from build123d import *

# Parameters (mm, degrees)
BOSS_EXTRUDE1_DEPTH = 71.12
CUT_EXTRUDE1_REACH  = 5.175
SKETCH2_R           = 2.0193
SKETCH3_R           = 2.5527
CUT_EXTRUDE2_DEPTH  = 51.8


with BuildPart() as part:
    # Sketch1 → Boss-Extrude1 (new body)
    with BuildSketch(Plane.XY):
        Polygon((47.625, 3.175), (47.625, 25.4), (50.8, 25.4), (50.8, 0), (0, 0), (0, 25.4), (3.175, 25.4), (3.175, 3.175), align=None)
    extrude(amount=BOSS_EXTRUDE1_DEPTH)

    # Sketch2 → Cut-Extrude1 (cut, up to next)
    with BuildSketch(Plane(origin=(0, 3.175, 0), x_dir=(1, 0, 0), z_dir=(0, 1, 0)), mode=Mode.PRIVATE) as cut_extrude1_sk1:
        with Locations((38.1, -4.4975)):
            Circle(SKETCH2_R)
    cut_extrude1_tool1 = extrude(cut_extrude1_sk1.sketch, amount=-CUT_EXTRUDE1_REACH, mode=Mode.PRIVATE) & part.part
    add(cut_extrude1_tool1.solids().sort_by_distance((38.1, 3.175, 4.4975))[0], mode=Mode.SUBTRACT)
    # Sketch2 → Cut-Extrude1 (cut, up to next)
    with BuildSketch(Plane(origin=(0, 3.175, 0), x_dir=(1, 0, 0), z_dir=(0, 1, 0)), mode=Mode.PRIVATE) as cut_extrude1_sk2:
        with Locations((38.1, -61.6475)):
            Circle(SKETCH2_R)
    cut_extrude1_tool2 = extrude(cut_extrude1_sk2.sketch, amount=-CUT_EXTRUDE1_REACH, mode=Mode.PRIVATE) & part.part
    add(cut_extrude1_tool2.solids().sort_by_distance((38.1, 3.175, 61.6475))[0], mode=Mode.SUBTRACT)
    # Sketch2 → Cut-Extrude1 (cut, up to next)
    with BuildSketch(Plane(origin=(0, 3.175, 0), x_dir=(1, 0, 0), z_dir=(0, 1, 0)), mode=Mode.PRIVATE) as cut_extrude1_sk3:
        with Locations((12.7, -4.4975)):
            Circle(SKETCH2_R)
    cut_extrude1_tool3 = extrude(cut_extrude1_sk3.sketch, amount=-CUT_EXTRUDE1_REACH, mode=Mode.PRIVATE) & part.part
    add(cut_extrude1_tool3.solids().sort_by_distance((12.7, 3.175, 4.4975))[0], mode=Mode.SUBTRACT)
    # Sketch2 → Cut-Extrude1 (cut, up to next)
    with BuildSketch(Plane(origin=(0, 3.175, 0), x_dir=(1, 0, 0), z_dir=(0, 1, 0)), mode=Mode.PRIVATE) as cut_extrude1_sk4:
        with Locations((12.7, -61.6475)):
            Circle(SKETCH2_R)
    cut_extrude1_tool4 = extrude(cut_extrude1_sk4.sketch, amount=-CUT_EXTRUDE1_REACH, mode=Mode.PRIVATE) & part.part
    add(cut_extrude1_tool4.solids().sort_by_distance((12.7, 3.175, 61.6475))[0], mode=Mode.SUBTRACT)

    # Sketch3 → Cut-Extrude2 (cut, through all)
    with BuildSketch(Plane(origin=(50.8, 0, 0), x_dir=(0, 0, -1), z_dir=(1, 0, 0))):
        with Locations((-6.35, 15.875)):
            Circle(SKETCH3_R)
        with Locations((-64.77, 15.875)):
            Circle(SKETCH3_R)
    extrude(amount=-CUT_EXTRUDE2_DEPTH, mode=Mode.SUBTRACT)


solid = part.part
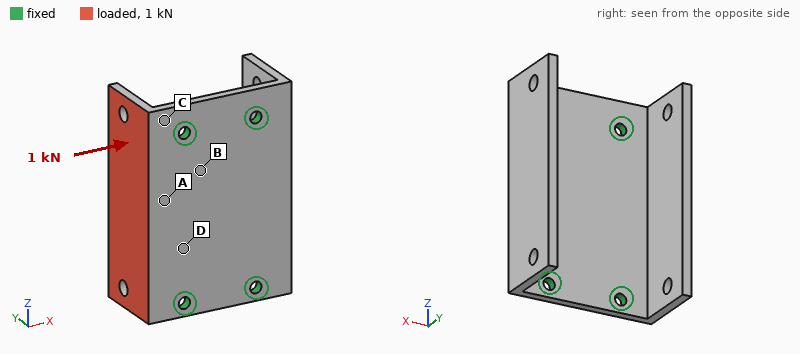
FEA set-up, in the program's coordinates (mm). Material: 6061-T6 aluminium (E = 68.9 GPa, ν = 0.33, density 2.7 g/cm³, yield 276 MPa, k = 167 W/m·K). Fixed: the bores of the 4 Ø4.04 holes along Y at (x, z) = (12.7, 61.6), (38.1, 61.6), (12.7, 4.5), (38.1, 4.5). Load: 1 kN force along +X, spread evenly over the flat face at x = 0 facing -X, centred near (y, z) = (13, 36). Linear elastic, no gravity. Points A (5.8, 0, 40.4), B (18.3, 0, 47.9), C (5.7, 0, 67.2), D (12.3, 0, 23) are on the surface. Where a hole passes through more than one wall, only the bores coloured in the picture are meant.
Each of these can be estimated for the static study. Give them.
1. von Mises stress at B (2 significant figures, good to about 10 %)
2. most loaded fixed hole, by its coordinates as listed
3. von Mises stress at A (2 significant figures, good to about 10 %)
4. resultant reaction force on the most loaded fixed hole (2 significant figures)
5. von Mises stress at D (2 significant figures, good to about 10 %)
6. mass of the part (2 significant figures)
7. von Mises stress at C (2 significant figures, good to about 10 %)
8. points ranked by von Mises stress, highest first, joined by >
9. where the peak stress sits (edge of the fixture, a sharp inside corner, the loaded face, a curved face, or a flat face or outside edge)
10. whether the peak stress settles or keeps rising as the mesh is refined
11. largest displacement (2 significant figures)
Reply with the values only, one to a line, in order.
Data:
25 MPa
(12.7, 61.6)
65 MPa
380 N
48 MPa
57 g
87 MPa
C > A > D > B
edge of the fixture
keeps rising
0.35 mm
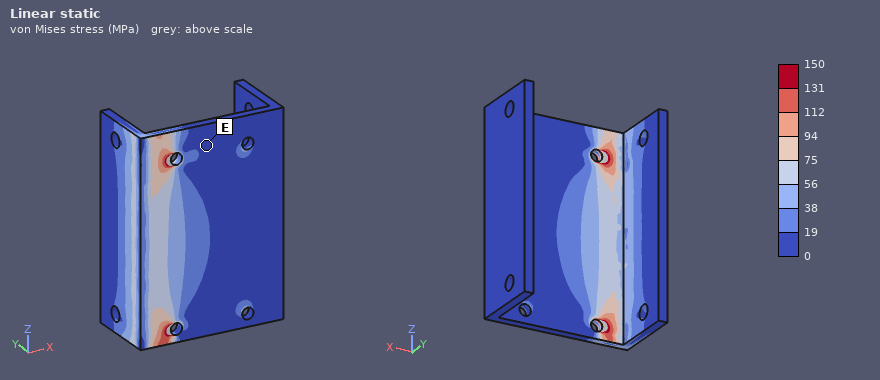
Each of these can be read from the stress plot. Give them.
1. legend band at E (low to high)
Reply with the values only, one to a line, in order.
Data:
0 to 19 MPa
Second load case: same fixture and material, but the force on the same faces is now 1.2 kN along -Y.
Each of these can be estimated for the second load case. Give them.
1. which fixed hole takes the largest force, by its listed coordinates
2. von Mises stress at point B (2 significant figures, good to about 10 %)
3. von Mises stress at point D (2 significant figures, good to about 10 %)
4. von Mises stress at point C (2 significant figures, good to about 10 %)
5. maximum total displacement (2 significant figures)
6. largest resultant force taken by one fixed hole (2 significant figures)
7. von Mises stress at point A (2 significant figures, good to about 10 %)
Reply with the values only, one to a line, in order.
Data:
(12.7, 61.6)
29 MPa
38 MPa
70 MPa
0.25 mm
760 N
36 MPa
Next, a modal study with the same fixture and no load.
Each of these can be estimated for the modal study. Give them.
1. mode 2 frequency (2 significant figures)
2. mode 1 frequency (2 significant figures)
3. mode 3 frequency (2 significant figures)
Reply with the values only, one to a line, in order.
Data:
2600 Hz
2500 Hz
4100 Hz
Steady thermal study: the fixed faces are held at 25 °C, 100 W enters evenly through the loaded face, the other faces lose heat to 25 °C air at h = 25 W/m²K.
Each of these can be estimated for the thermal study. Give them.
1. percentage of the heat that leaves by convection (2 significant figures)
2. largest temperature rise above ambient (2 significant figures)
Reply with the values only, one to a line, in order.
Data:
6.4 %
74 K
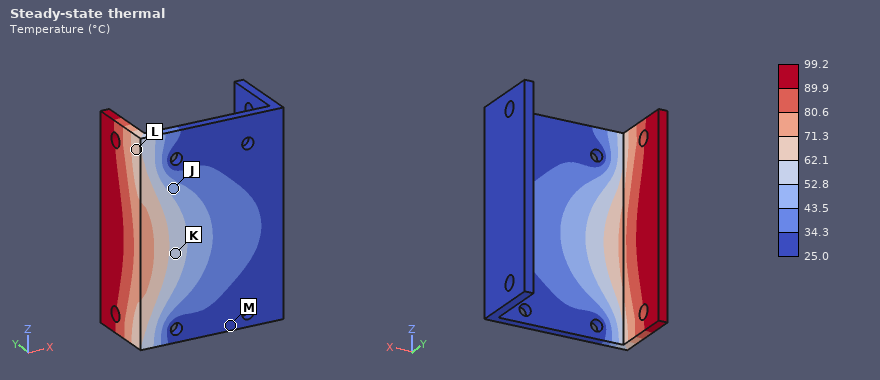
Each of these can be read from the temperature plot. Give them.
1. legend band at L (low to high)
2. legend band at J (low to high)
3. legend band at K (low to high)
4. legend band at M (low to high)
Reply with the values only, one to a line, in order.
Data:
62.1 to 71.3 °C
43.5 to 52.8 °C
52.8 to 62.1 °C
25.0 to 34.3 °C
